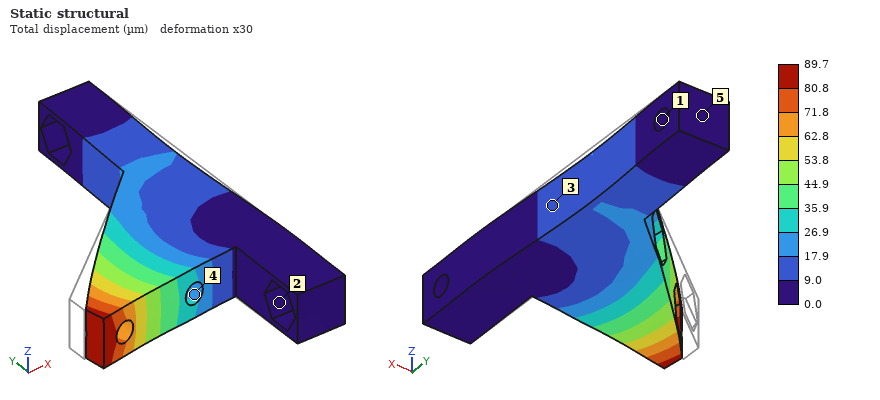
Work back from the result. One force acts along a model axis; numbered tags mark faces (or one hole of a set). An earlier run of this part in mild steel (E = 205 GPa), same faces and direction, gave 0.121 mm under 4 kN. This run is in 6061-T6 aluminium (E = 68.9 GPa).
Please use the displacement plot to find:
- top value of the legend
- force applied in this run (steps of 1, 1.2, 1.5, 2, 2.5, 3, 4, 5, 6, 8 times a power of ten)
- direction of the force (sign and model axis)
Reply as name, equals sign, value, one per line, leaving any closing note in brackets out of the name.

top value of the legend = 89.7 µm
force applied in this run = 1 kN
direction of the force = -Y
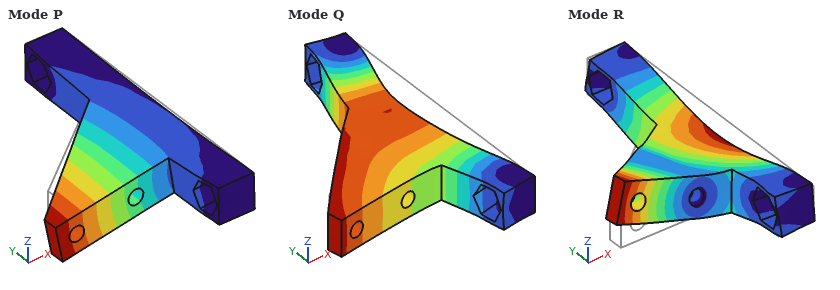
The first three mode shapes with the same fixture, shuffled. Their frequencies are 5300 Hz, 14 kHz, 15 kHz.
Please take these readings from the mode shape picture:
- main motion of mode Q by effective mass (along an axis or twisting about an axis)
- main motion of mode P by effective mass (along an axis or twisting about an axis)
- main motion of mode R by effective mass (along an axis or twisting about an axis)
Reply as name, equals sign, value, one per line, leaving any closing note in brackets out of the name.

main motion of mode Q by effective mass = along X
main motion of mode P by effective mass = along Z
main motion of mode R by effective mass = along Z
